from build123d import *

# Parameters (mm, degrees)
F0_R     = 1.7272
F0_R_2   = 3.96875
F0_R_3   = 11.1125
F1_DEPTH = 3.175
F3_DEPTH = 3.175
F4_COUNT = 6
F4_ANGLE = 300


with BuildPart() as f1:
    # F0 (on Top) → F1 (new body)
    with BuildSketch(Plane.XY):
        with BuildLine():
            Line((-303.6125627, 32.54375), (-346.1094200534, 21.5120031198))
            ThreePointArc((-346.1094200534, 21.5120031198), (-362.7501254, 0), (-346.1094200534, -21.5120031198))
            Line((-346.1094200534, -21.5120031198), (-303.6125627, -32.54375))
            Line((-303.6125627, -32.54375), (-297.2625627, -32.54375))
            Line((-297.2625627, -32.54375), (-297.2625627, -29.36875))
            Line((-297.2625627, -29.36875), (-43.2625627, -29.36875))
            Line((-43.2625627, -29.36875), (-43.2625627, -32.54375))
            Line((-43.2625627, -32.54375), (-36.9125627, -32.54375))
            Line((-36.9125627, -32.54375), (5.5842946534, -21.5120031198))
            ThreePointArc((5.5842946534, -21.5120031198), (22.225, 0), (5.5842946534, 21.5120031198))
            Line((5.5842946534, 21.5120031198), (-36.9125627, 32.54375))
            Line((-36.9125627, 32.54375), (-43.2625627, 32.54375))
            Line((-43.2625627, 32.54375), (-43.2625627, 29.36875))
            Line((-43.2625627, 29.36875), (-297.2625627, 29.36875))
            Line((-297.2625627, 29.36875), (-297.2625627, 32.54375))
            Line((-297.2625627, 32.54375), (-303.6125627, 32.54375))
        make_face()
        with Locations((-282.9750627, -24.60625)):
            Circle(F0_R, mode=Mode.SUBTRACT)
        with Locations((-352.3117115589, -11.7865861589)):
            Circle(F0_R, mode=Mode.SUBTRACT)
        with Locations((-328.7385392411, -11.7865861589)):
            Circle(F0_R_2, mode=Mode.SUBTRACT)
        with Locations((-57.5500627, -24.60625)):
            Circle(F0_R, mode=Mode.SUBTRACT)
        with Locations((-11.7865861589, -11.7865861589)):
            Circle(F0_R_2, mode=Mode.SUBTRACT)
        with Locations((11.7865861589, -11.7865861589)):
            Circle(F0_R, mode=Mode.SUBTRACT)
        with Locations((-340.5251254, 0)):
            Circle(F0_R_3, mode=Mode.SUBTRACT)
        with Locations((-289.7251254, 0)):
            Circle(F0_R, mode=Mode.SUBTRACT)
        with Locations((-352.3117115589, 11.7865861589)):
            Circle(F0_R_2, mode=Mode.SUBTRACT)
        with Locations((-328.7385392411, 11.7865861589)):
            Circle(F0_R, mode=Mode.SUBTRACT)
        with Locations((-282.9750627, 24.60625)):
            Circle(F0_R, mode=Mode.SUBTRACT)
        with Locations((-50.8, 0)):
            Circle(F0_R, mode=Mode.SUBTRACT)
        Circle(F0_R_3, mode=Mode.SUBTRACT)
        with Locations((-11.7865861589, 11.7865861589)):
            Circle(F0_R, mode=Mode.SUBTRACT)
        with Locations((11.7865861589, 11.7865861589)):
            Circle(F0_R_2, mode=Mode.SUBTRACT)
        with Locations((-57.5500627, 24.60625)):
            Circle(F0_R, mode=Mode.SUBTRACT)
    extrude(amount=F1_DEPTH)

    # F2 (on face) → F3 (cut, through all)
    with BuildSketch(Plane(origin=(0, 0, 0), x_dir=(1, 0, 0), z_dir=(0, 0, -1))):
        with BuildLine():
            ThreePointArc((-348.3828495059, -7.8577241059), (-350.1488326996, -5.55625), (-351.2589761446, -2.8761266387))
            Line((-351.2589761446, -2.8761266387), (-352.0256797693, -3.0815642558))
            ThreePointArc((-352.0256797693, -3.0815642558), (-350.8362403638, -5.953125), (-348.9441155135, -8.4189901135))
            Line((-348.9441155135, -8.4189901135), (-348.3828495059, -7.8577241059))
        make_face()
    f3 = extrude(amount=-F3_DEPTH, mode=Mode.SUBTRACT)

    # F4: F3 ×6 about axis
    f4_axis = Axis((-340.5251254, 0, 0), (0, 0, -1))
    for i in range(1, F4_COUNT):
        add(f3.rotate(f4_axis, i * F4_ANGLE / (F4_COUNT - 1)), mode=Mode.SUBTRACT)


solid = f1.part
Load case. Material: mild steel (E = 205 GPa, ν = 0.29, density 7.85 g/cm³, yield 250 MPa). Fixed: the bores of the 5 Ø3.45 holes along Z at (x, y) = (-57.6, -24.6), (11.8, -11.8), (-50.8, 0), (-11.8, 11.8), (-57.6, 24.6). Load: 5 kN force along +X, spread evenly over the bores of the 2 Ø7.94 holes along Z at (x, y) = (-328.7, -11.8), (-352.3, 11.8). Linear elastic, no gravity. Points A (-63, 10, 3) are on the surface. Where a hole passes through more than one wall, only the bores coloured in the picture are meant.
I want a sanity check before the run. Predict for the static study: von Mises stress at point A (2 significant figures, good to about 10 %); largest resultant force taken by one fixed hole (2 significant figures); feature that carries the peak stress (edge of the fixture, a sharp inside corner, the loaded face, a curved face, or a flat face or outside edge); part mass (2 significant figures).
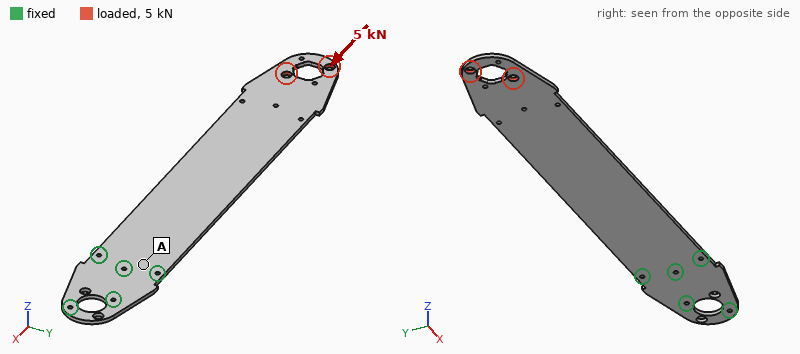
18 MPa
1.6 kN
the loaded face
510 g
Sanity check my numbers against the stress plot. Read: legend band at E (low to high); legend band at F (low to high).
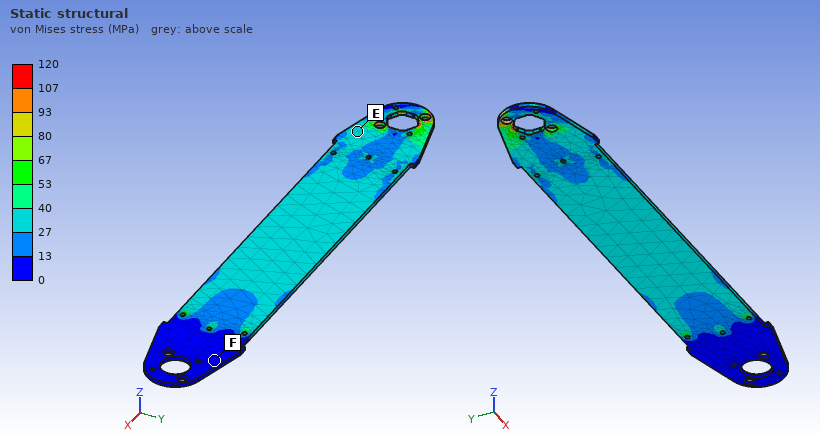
27 to 40 MPa
0 to 13 MPa
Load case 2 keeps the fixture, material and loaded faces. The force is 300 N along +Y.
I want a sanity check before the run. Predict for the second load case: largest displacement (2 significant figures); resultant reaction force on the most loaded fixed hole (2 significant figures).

0.24 mm
1.6 kN
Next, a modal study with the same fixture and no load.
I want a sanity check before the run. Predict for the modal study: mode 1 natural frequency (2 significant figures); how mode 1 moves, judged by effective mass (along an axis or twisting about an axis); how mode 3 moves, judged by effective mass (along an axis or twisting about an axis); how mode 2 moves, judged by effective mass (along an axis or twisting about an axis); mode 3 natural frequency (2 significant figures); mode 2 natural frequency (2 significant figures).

32 Hz
along Z
twisting about X
along Z
320 Hz
190 Hz
